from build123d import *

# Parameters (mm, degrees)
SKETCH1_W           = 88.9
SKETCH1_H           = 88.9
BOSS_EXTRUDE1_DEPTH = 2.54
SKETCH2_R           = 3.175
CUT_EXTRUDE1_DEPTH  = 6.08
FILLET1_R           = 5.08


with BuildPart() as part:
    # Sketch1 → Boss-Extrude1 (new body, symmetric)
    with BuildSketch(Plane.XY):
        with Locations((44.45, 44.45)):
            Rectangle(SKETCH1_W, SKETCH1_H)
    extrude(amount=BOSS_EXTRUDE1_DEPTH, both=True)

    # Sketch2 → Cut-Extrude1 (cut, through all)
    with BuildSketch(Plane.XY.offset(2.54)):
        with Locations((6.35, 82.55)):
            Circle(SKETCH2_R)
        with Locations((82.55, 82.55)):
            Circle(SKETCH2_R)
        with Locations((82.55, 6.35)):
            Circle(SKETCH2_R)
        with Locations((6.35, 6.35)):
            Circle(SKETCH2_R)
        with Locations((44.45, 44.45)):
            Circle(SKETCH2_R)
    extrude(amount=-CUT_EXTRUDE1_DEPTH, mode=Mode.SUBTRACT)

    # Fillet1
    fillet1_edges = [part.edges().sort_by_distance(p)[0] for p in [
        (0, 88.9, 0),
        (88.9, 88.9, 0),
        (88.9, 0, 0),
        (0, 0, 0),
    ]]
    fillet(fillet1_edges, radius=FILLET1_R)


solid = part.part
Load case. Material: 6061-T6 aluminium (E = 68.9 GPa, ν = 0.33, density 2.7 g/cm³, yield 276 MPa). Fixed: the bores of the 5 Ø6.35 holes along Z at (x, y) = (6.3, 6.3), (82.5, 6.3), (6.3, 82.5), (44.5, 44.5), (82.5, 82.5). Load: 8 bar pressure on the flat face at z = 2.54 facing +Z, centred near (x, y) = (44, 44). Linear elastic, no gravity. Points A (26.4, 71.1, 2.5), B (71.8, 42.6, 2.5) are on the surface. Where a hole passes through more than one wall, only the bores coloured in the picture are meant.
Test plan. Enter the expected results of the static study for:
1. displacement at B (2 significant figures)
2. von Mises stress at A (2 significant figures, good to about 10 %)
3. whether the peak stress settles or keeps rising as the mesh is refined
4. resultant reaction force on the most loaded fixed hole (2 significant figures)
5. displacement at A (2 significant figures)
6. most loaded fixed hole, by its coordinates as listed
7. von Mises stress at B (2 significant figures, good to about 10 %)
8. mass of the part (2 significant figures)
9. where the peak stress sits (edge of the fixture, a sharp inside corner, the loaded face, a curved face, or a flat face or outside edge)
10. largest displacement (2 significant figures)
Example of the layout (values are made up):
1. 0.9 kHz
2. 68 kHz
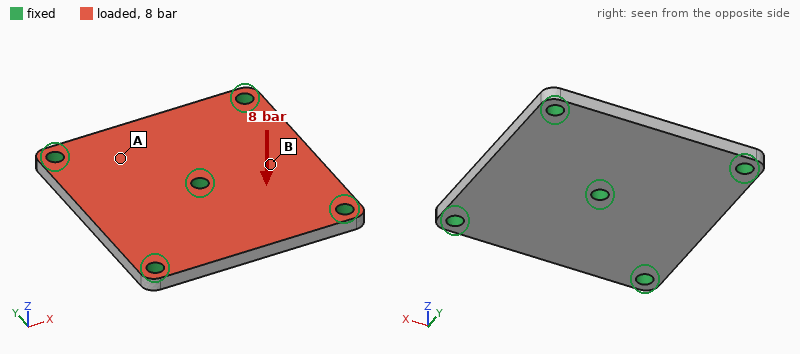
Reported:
1. 42 µm
2. 28 MPa
3. keeps rising
4. 2.4 kN
5. 34 µm
6. (44.5, 44.5)
7. 12 MPa
8. 110 g
9. edge of the fixture
10. 61 µm
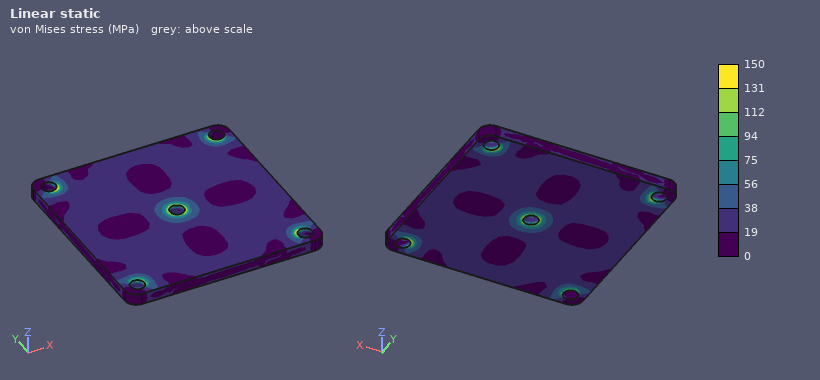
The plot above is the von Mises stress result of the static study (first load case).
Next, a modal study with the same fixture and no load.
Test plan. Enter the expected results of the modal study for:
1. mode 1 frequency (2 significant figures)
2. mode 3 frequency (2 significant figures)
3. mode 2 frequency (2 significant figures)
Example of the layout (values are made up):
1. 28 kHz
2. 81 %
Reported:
1. 5600 Hz
2. 5800 Hz
3. 5800 Hz
